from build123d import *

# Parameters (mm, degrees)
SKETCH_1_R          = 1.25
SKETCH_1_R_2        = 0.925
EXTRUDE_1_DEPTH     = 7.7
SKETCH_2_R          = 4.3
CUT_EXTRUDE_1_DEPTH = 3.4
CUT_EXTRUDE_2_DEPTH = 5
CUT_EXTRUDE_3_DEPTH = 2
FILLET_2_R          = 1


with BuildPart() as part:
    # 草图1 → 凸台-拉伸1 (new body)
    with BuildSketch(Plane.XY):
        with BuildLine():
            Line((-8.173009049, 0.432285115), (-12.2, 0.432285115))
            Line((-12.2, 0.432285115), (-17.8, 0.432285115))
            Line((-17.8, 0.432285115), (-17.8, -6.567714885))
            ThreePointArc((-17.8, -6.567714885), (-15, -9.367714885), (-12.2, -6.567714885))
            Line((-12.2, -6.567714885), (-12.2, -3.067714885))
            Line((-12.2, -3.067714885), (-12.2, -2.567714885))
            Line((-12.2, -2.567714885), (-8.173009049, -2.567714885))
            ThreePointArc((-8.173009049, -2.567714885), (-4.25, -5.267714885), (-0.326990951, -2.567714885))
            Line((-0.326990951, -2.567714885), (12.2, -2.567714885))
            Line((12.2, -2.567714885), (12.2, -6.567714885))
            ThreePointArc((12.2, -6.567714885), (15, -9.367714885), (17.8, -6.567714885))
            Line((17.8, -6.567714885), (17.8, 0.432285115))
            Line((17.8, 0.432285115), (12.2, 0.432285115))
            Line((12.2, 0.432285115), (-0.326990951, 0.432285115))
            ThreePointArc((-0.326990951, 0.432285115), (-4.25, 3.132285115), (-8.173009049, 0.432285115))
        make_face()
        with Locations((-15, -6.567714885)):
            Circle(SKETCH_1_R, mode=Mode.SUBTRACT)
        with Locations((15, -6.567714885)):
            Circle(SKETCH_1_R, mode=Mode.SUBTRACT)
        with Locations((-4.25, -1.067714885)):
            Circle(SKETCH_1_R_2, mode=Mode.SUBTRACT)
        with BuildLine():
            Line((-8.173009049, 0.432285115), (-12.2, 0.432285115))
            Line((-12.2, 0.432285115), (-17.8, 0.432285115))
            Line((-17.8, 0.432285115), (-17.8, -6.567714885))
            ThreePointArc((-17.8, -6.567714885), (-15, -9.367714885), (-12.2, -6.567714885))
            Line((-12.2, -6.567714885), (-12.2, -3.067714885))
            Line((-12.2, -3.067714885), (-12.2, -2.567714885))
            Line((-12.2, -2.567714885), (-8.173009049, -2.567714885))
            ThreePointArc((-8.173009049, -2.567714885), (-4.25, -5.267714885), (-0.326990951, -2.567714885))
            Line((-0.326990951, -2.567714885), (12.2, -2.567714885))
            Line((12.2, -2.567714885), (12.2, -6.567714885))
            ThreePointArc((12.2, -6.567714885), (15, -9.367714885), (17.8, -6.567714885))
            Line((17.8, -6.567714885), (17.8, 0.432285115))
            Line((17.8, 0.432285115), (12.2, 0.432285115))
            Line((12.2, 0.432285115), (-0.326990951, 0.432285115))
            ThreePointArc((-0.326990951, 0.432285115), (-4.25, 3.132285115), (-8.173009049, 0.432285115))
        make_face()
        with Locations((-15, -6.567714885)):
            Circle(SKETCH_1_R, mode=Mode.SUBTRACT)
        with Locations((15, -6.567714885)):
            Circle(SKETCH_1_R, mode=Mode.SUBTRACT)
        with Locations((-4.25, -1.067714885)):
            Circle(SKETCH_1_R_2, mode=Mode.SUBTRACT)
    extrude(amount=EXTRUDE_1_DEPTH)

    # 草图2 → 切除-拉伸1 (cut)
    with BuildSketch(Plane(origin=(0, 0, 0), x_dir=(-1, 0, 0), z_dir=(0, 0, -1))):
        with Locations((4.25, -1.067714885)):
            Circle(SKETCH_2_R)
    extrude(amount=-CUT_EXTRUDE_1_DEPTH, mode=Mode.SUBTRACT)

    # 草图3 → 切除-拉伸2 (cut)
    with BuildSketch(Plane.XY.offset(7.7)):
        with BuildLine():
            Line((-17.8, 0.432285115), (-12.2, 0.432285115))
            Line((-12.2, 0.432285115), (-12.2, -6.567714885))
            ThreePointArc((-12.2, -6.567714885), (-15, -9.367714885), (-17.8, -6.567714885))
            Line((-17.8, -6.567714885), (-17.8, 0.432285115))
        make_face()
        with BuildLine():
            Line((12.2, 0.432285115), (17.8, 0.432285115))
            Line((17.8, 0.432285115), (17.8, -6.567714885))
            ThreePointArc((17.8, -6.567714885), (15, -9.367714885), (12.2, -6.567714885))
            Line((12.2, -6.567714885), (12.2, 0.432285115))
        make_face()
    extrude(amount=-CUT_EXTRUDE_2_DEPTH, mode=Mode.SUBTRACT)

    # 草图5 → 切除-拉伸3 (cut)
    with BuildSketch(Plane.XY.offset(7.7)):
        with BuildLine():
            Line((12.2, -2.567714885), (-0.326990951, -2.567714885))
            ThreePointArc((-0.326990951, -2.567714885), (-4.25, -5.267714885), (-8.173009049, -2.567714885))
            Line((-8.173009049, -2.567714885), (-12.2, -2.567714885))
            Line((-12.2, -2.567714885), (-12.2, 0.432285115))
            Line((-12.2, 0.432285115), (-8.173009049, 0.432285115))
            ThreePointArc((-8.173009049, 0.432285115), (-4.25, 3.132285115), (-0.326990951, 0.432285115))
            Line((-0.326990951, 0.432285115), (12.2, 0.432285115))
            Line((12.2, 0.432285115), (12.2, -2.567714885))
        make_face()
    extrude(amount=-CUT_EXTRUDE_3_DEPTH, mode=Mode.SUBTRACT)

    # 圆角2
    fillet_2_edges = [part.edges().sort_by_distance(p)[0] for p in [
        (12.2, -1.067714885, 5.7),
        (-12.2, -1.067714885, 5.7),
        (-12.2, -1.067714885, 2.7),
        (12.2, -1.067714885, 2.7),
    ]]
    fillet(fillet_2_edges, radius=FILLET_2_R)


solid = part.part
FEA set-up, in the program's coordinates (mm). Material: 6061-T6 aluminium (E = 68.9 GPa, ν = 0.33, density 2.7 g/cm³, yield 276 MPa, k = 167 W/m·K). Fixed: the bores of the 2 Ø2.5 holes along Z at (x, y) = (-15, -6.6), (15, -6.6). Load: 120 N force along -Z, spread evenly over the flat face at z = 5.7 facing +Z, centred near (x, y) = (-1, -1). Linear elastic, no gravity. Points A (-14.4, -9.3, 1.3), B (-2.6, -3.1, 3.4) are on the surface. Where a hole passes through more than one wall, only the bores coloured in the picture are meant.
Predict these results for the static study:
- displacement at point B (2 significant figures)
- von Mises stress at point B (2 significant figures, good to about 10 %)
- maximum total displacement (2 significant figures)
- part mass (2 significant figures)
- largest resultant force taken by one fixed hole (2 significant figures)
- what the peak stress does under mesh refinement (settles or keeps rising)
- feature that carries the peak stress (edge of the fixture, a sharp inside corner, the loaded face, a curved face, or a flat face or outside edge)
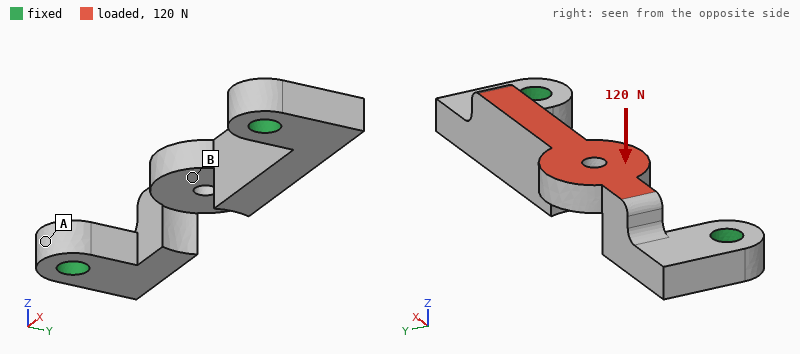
24 µm
18 MPa
33 µm
1.7 g
100 N
keeps rising
a sharp inside corner
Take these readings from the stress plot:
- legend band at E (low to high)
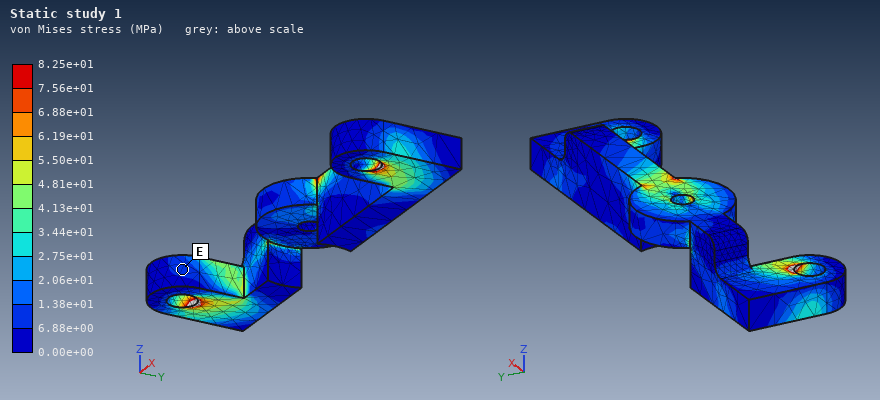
6.88e+00 to 1.38e+01 MPa
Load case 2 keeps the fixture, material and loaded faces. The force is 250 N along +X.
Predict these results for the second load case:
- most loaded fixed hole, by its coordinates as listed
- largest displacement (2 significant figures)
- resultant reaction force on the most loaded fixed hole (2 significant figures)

(15, -6.6)
10 µm
150 N
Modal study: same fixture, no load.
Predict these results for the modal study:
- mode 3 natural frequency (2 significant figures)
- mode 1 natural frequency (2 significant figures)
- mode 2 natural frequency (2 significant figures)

23 kHz
11 kHz
16 kHz
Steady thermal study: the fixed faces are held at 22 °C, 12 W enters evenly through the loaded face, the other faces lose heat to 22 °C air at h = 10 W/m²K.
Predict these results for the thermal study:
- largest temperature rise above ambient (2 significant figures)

41 K
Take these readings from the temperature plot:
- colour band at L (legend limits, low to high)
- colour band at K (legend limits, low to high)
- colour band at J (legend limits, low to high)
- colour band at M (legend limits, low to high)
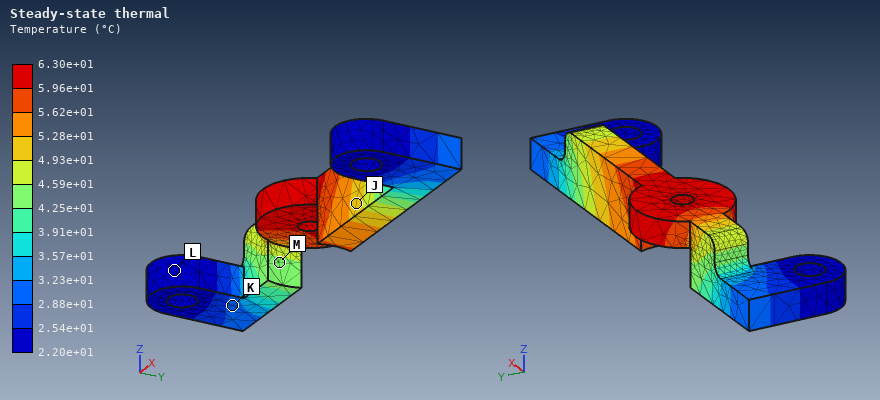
2.20e+01 to 2.54e+01 °C
2.88e+01 to 3.23e+01 °C
4.93e+01 to 5.28e+01 °C
4.25e+01 to 4.59e+01 °C
